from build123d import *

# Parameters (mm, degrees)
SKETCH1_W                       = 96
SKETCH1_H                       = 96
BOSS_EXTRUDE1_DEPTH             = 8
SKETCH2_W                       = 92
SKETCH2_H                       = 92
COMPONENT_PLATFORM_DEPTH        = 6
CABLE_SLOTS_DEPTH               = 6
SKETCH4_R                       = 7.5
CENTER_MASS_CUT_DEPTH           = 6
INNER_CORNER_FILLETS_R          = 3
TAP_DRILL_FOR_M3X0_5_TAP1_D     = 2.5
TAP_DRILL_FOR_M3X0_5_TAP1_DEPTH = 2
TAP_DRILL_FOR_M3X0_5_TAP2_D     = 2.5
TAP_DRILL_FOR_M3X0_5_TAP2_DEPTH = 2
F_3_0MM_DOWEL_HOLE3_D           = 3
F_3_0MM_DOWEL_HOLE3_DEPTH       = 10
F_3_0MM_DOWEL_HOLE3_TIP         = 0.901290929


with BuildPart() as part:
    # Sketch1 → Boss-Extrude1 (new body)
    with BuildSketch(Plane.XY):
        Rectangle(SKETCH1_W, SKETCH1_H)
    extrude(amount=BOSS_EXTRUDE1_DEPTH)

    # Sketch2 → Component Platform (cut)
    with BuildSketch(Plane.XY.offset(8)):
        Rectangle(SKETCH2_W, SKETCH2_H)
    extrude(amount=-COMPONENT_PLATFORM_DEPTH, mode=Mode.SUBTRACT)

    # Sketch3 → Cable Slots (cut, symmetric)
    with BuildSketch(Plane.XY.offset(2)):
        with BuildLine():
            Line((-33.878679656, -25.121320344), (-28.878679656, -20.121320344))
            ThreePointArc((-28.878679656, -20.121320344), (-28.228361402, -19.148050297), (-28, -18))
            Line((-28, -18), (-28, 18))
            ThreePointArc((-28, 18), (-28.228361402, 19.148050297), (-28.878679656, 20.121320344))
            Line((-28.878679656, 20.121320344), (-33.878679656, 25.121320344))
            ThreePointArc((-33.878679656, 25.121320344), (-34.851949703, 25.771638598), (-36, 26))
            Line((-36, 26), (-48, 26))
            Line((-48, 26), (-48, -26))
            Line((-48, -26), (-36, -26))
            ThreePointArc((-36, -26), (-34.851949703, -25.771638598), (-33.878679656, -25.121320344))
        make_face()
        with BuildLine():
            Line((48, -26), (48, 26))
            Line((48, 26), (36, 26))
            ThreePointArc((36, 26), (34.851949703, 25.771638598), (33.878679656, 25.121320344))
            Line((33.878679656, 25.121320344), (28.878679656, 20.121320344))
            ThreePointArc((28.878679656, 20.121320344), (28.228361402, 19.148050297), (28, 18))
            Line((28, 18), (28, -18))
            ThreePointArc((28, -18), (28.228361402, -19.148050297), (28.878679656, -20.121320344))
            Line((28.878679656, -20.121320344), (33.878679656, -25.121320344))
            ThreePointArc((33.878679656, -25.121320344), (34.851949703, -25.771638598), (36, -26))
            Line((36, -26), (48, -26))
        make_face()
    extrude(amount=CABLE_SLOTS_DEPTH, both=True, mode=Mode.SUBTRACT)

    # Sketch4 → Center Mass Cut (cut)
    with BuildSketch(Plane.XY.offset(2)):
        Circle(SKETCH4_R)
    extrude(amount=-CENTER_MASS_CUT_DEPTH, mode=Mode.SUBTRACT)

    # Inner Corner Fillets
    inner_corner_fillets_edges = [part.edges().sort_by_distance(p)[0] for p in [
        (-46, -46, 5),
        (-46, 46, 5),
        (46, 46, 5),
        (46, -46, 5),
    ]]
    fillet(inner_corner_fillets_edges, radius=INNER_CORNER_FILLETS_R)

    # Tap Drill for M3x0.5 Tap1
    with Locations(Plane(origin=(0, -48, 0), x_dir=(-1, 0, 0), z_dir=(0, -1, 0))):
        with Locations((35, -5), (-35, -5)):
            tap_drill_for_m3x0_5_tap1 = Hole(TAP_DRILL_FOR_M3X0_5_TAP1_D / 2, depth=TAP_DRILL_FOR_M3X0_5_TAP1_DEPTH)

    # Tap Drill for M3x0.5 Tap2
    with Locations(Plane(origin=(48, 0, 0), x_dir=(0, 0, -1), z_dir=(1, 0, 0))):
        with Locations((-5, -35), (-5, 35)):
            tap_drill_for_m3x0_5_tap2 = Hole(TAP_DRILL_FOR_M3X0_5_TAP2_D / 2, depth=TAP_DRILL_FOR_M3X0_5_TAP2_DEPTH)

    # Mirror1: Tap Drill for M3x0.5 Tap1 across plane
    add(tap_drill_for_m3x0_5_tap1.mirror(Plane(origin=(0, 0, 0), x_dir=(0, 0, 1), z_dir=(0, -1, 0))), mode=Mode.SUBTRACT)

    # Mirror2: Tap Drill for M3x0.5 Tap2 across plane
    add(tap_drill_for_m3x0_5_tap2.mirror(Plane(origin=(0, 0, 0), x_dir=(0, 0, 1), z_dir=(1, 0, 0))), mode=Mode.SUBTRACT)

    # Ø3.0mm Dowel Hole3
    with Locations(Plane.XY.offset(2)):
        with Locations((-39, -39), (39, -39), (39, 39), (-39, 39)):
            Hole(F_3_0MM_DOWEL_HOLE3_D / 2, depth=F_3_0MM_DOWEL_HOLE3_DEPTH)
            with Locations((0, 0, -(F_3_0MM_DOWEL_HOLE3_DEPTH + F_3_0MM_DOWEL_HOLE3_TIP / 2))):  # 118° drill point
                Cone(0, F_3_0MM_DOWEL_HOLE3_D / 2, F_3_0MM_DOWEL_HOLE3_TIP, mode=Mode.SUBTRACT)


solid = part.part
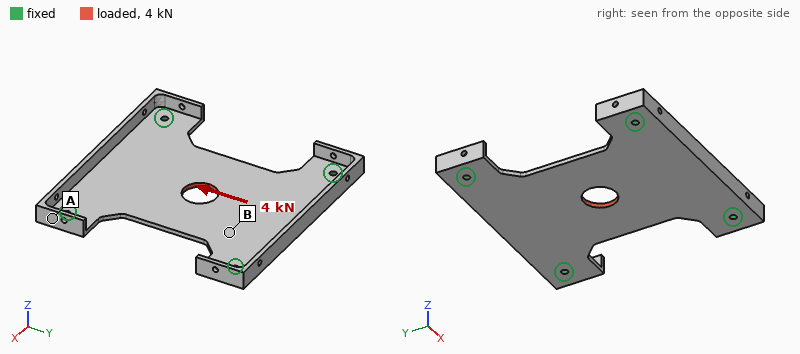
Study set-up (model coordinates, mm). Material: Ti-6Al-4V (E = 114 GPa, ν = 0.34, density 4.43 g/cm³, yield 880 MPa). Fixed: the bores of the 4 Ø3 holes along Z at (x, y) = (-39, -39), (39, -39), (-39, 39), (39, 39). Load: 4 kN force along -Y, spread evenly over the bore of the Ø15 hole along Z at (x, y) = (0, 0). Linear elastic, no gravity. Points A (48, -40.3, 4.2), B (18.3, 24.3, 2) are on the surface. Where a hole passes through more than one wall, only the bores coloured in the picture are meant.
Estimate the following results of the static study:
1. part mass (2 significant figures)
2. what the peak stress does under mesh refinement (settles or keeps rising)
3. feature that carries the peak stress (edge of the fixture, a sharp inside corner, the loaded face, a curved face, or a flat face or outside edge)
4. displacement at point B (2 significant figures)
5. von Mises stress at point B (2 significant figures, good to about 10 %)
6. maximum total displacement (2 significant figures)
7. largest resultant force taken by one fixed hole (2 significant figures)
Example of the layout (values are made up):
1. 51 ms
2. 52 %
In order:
1. 77 g
2. keeps rising
3. edge of the fixture
4. 17 µm
5. 30 MPa
6. 30 µm
7. 1.1 kN
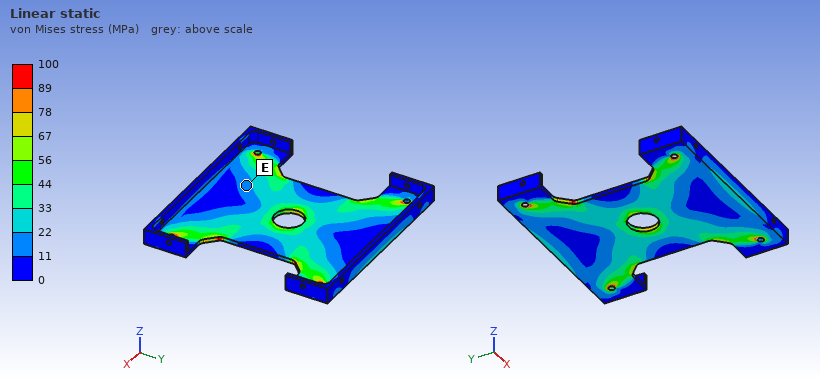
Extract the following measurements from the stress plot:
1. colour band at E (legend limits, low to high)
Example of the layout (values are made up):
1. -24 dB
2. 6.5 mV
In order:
1. 11 to 22 MPa
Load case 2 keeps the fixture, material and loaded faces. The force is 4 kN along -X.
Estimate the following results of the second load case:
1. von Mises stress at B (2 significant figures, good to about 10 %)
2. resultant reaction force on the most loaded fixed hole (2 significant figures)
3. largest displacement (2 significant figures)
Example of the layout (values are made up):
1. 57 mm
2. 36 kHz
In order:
1. 29 MPa
2. 1.2 kN
3. 21 µm
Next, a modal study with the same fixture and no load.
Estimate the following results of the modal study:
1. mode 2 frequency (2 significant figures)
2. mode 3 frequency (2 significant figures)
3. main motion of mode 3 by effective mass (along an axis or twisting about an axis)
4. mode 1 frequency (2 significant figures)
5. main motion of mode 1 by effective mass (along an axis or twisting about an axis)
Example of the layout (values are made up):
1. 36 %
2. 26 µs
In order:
1. 2400 Hz
2. 2600 Hz
3. twisting about X
4. 1200 Hz
5. along Z
